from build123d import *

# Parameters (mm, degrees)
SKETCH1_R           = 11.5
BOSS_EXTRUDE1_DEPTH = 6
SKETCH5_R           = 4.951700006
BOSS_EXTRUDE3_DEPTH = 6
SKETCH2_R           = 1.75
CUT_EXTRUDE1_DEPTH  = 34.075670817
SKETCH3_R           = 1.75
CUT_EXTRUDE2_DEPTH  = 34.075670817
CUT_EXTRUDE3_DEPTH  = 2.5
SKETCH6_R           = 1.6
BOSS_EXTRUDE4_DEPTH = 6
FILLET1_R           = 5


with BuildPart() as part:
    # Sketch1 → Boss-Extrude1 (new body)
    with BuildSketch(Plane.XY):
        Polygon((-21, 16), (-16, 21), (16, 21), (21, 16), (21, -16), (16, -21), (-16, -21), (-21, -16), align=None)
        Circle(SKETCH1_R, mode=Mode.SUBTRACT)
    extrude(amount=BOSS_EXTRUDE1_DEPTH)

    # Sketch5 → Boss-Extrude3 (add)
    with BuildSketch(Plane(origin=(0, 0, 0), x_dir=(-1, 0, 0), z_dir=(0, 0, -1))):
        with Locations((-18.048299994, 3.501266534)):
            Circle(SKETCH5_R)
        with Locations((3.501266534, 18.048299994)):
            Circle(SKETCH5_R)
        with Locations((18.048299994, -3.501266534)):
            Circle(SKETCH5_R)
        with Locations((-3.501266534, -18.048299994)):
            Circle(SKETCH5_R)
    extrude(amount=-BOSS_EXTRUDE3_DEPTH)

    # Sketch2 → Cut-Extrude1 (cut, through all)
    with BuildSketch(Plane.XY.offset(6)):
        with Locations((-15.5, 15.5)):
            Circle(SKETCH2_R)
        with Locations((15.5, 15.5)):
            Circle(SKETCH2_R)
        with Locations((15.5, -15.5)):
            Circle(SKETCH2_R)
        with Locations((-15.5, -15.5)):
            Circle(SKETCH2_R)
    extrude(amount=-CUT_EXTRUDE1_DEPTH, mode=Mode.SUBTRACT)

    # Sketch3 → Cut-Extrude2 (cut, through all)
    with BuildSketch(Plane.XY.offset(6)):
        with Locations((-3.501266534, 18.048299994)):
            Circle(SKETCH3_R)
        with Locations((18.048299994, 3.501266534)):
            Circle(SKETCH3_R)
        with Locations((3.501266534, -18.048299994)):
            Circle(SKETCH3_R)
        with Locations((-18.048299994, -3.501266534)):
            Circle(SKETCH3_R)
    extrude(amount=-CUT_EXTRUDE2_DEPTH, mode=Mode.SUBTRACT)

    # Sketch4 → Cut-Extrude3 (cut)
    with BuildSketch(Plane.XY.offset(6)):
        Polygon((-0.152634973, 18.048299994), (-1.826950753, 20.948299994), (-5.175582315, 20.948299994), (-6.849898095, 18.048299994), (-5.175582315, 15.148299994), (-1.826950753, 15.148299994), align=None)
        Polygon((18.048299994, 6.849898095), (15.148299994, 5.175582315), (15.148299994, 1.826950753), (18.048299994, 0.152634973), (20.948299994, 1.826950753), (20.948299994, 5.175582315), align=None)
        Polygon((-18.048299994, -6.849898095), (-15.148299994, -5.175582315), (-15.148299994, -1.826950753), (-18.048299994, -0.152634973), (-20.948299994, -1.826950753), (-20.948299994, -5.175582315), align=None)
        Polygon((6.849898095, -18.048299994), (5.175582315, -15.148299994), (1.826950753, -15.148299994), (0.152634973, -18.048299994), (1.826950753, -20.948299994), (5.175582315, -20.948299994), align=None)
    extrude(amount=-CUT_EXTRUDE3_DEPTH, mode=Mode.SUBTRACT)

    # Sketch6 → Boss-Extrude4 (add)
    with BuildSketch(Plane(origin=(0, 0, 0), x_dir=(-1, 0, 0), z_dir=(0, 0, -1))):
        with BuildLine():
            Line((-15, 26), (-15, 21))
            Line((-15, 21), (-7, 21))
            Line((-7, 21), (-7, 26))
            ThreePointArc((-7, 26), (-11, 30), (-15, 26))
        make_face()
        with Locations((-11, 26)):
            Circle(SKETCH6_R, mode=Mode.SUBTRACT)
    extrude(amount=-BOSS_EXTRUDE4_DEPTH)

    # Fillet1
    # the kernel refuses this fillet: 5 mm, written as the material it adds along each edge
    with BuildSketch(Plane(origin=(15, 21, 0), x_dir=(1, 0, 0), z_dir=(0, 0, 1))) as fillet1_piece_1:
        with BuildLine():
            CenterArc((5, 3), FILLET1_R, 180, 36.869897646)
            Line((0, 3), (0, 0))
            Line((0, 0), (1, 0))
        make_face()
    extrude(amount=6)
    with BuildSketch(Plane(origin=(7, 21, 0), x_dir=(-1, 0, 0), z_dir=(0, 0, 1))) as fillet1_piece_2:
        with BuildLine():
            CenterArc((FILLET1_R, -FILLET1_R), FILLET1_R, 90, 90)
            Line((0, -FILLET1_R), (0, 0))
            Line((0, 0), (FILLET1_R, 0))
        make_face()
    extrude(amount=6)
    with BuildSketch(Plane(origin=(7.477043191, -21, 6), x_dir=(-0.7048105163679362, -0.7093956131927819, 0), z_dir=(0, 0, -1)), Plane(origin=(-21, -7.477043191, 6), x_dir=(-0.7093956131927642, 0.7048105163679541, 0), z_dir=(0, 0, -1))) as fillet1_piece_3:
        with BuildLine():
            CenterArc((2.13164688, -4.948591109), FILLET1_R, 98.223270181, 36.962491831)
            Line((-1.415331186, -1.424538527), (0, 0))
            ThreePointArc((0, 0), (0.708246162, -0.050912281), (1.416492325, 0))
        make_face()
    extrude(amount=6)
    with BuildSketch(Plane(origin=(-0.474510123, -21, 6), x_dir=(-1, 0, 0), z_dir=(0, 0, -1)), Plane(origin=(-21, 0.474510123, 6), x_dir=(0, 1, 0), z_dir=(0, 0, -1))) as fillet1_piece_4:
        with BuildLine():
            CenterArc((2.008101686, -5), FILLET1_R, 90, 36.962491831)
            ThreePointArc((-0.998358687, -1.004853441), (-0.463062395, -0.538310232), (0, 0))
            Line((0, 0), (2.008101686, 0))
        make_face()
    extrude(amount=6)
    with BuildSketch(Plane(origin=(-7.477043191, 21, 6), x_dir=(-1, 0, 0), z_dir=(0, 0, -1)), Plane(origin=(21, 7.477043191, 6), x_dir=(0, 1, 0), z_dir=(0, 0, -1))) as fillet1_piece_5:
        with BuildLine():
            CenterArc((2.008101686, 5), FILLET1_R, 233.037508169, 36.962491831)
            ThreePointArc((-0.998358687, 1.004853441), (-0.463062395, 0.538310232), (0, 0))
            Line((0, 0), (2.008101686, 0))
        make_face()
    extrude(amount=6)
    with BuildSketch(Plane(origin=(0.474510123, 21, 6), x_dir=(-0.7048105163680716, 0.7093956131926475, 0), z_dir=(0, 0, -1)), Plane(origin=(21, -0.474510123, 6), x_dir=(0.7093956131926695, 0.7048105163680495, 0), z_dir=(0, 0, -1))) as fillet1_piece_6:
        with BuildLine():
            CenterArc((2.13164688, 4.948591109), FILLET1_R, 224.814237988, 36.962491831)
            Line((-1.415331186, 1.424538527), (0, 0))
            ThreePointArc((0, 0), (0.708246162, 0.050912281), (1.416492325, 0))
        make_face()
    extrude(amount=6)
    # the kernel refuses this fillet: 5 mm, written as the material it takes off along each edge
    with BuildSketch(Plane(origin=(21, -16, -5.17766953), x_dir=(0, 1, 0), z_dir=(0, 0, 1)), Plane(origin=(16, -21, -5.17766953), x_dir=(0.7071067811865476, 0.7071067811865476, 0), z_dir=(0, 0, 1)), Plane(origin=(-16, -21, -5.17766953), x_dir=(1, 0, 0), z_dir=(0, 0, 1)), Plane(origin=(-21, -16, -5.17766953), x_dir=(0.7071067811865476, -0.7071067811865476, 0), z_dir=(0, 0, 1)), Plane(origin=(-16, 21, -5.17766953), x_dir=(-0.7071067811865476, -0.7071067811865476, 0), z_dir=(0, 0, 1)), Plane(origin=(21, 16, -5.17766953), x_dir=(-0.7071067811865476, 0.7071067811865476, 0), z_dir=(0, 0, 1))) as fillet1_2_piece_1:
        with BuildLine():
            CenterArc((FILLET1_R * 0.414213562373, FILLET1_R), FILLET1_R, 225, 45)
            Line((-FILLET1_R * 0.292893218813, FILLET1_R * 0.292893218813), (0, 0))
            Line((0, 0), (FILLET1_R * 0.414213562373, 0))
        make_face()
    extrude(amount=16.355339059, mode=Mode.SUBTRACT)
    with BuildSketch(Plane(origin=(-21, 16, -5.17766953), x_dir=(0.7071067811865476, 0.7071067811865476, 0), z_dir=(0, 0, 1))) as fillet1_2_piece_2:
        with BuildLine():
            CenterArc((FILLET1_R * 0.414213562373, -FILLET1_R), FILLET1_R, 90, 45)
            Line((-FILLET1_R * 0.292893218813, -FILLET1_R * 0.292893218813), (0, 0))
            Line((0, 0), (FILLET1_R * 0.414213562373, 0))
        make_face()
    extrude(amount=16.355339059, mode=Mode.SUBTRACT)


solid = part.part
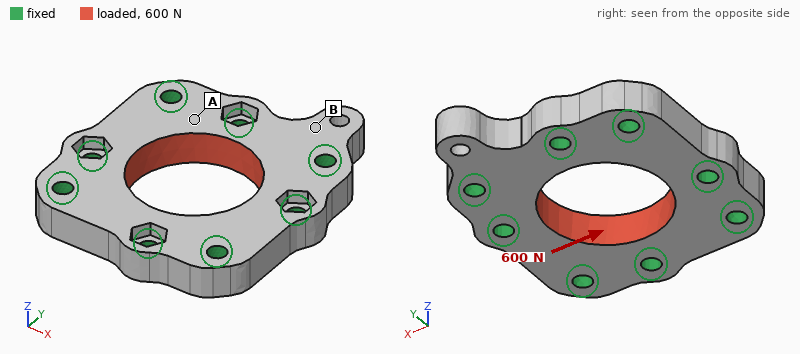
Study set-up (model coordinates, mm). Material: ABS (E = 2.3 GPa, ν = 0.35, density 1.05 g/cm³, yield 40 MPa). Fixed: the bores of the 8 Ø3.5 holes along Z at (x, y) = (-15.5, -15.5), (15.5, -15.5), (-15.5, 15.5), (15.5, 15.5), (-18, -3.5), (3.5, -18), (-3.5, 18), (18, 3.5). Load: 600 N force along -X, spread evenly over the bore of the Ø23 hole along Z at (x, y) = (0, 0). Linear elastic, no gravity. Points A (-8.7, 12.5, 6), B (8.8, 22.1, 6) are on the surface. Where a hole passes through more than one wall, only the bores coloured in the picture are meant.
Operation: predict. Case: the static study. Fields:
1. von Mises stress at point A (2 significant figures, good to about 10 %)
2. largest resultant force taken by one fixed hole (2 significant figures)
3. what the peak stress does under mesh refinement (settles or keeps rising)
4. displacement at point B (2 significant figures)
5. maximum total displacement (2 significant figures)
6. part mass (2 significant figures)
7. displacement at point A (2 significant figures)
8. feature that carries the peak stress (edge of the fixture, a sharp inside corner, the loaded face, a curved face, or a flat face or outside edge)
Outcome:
1.4 MPa
110 N
keeps rising
2.4 µm
14 µm
8.2 g
4.7 µm
edge of the fixture
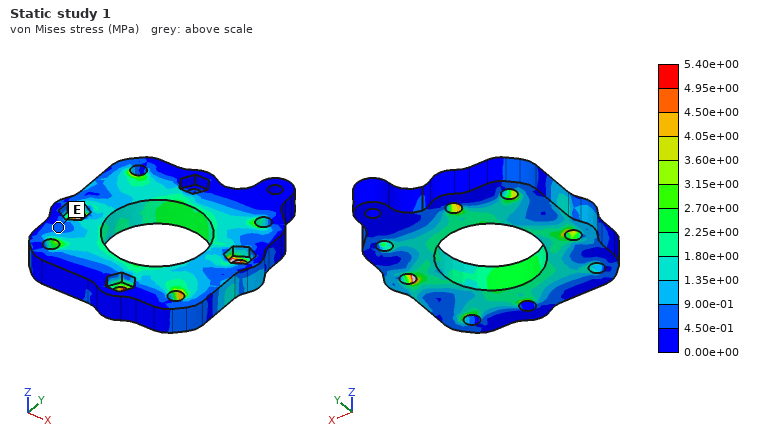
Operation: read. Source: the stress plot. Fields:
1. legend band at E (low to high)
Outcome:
4.50e-01 to 9.00e-01 MPa
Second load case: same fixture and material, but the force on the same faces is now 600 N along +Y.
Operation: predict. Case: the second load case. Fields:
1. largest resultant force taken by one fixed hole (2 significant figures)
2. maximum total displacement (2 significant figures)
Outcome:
110 N
14 µm
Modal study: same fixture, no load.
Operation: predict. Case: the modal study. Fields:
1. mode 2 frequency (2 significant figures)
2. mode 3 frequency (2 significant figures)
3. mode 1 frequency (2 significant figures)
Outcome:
13 kHz
14 kHz
8100 Hz
